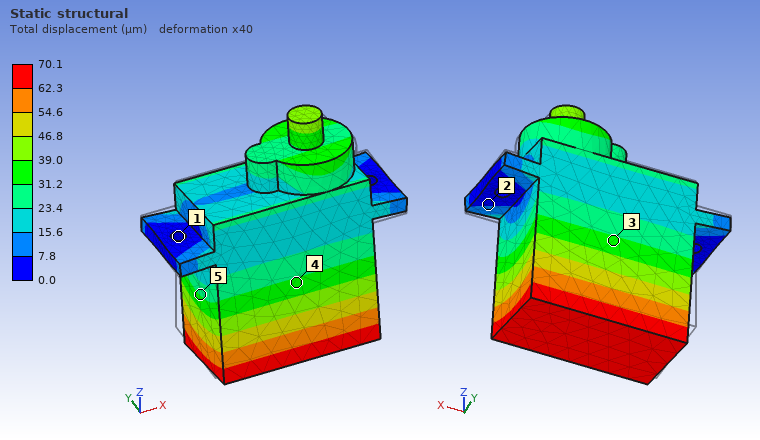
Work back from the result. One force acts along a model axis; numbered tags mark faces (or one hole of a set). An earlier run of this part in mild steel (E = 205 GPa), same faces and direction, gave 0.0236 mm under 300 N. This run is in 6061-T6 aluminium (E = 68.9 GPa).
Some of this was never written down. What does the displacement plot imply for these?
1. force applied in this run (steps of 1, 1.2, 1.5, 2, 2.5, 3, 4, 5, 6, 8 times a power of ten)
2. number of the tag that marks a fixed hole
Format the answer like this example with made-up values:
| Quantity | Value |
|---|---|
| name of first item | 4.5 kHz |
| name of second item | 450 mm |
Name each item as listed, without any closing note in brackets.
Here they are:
| Quantity | Value |
|---|---|
| force applied in this run | 300 N |
| number of the tag that marks a fixed hole | 1 |
